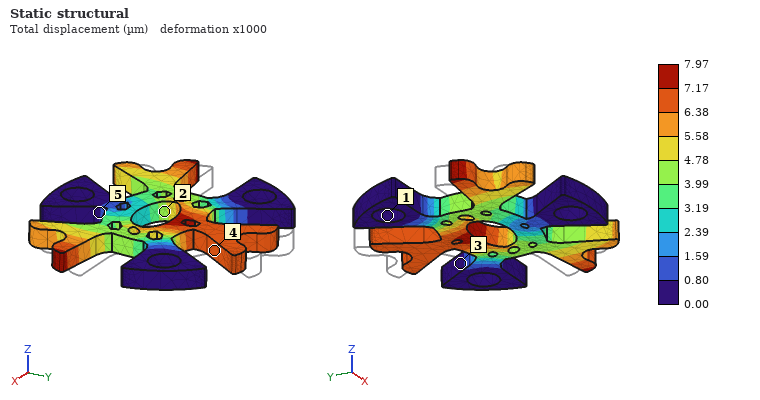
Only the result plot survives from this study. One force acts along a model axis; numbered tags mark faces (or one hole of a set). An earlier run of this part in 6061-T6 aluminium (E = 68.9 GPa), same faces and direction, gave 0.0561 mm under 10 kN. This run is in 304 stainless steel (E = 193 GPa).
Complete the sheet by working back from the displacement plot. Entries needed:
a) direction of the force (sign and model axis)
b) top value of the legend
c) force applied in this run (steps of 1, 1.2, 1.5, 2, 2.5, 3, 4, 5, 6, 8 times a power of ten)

-Y
7.97 µm
4 kN
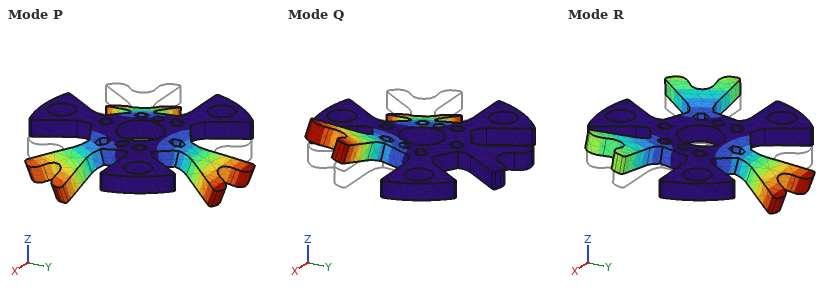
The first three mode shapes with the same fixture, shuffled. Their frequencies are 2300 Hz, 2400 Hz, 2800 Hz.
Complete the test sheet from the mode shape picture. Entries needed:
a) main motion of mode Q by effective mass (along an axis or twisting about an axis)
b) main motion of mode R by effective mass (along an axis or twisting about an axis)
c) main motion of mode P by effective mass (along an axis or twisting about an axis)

twisting about Y
twisting about X
along Z
